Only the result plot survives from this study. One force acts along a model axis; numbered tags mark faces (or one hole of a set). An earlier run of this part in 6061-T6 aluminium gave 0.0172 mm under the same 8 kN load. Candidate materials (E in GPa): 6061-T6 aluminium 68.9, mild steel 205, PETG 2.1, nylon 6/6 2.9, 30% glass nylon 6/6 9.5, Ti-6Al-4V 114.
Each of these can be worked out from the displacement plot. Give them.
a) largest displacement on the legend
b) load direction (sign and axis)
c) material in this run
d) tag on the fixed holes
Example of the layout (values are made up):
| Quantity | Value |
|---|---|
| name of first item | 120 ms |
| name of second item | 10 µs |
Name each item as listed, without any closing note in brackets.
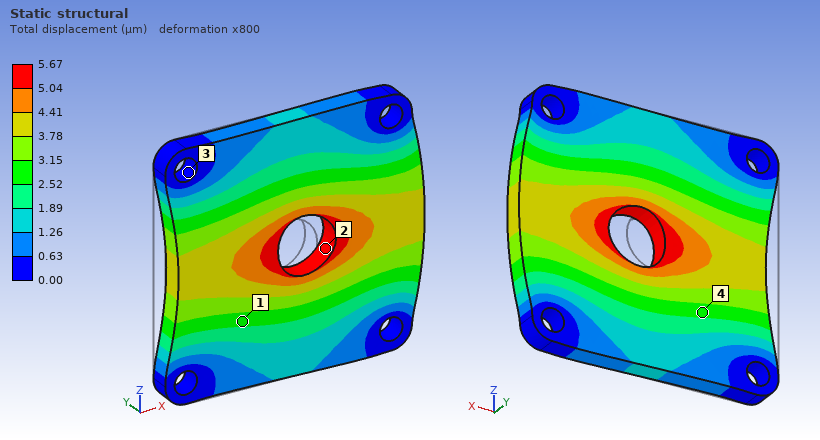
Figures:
| Quantity | Value |
|---|---|
| largest displacement on the legend | 5.67 µm |
| load direction | +X |
| material in this run | mild steel |
| tag on the fixed holes | 3 |
